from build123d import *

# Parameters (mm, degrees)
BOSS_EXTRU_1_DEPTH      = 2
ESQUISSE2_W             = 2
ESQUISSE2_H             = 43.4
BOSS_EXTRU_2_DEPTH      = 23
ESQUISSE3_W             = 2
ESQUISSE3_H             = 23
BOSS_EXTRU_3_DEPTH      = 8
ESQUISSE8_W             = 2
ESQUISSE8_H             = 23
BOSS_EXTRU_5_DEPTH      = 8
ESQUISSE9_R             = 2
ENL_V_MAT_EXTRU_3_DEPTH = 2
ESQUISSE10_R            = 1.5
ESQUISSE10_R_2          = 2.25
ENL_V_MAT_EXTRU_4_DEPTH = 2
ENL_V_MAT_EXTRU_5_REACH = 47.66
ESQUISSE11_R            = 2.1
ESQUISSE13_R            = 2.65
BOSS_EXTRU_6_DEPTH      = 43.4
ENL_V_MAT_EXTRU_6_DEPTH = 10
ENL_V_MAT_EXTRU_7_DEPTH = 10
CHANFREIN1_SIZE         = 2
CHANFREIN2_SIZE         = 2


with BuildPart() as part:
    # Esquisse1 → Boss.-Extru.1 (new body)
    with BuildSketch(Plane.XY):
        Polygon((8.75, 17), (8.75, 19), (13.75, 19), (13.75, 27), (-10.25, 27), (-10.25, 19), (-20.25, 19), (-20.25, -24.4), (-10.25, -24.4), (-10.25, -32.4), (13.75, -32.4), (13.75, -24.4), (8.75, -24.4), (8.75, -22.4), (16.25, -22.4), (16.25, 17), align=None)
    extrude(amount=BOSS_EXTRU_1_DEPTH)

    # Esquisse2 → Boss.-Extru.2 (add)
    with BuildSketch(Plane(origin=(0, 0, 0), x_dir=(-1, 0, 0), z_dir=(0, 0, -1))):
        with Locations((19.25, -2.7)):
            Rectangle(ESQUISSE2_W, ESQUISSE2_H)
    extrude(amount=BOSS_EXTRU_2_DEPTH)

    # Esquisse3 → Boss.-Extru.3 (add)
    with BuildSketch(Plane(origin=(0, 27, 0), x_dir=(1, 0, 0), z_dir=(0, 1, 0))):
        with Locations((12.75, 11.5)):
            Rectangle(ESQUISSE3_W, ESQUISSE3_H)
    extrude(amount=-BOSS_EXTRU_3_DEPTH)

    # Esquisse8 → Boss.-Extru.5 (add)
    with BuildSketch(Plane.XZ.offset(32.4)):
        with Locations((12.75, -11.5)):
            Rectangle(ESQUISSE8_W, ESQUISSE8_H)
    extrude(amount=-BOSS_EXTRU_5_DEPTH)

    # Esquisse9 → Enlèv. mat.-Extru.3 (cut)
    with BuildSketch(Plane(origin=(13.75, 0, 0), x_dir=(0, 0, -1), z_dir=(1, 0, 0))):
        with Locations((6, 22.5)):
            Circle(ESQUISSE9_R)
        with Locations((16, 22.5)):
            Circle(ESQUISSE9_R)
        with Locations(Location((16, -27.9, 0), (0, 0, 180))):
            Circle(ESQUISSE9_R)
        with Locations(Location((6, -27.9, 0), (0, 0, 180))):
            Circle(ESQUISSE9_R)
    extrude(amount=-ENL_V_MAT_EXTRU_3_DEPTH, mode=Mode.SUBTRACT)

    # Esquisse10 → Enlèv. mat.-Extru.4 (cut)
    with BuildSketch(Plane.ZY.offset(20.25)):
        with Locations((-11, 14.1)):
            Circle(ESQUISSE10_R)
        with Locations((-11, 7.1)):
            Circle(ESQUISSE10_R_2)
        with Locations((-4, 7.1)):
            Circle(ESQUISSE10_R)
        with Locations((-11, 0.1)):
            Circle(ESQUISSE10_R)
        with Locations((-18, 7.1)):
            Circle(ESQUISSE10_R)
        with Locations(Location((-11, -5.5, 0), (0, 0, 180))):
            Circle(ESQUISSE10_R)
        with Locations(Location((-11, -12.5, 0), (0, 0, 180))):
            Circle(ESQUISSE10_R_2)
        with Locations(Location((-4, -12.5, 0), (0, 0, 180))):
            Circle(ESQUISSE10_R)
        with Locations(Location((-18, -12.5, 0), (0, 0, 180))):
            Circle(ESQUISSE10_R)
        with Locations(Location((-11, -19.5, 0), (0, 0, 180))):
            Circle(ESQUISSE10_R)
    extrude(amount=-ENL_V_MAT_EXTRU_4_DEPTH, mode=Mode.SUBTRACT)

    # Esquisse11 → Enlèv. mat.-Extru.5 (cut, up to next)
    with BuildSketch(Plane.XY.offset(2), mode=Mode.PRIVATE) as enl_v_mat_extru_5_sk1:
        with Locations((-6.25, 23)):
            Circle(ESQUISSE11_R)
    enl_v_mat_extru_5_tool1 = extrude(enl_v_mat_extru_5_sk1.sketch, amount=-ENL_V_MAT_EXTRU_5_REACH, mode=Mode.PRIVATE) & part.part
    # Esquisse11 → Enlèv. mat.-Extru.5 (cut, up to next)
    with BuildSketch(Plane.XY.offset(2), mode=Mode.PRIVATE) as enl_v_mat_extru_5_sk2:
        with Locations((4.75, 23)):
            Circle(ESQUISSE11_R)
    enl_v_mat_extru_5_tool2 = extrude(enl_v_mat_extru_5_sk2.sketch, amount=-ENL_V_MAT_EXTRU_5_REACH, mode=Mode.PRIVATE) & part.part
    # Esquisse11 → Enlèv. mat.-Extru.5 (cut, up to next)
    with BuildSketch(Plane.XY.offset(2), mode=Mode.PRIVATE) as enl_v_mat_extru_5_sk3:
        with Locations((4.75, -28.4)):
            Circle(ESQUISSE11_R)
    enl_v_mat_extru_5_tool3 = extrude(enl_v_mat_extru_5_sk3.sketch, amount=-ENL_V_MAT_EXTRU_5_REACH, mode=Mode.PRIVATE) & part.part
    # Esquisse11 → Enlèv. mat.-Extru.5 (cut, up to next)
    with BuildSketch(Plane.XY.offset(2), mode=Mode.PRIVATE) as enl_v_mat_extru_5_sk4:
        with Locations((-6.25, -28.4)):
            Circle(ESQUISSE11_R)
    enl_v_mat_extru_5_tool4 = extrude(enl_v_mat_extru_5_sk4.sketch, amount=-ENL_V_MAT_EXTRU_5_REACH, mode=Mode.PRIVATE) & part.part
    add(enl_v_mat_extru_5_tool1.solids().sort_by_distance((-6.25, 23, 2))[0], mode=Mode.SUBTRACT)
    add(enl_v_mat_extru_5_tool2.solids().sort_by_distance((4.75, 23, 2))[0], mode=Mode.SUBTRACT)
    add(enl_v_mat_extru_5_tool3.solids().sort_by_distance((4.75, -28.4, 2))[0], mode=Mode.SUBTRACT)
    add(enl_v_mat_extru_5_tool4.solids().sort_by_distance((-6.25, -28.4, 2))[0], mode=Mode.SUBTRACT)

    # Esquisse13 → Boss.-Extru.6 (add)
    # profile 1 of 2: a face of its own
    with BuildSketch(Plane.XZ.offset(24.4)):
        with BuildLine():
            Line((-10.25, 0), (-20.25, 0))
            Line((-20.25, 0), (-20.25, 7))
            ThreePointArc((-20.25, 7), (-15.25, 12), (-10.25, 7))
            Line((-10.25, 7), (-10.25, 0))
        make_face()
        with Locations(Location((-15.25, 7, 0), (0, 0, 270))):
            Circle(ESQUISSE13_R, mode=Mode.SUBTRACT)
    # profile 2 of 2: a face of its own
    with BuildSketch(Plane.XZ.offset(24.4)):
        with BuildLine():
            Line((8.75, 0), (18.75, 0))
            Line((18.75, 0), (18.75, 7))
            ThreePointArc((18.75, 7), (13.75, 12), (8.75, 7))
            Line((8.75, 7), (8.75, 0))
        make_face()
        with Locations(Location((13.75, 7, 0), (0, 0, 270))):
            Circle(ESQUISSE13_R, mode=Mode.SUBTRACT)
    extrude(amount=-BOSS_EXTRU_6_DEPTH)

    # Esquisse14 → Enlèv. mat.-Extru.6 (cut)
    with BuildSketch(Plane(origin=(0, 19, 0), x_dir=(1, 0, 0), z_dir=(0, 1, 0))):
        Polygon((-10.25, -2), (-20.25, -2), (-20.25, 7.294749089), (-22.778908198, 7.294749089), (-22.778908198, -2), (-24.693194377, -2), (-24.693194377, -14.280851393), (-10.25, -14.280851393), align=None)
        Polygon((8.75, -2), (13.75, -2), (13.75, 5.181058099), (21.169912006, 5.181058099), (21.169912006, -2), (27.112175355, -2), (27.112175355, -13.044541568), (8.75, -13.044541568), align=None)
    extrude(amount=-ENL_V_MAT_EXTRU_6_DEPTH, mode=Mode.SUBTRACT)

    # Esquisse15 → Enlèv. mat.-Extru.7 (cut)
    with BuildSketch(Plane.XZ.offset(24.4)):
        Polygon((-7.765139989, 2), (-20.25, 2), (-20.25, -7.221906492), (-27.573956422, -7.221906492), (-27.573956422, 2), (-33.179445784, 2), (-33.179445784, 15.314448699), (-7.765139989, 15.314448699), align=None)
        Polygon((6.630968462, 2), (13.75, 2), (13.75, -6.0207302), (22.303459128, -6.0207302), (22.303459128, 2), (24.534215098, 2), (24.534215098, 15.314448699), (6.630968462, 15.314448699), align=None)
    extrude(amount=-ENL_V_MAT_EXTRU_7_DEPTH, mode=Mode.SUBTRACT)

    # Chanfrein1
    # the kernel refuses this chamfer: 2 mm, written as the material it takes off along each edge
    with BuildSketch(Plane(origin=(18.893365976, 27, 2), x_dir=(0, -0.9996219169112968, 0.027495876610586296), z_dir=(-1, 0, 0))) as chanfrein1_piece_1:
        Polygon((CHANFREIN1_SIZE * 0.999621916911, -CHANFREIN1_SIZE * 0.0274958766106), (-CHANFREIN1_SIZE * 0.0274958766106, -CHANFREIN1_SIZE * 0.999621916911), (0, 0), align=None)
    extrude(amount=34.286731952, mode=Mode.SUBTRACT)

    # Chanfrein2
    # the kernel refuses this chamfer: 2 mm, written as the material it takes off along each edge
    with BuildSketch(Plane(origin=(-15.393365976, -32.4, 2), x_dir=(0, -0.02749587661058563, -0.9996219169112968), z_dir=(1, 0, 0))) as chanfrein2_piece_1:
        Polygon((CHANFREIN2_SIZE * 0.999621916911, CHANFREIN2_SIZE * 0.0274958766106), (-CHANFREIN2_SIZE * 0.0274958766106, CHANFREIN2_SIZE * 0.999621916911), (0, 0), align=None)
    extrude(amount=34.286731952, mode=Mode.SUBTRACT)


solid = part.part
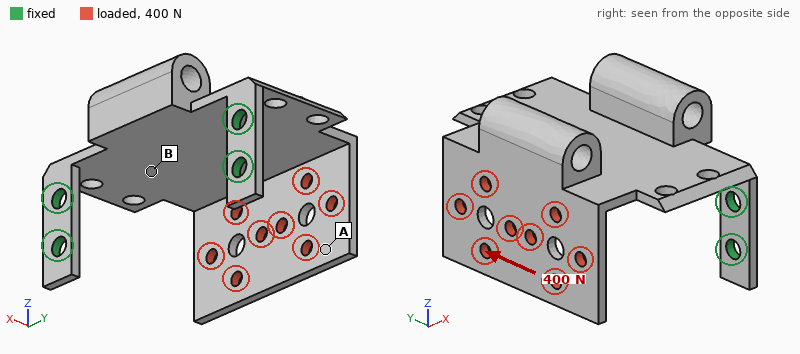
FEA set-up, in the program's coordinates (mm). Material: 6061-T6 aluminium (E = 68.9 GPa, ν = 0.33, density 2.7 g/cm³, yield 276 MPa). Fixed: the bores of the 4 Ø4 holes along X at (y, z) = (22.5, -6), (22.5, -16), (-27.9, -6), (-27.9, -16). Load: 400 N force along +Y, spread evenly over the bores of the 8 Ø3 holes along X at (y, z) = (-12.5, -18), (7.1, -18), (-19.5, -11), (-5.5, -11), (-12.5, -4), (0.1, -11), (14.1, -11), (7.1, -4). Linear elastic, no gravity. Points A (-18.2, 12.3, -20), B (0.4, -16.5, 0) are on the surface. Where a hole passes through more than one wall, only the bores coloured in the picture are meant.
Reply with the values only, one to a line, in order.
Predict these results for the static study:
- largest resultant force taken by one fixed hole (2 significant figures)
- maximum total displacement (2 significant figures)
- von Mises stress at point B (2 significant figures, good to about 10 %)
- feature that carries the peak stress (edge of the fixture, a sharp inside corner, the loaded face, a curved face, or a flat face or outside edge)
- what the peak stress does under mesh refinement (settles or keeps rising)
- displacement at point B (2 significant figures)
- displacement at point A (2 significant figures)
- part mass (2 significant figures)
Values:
360 N
0.65 mm
60 MPa
edge of the fixture
keeps rising
0.13 mm
0.54 mm
25 g
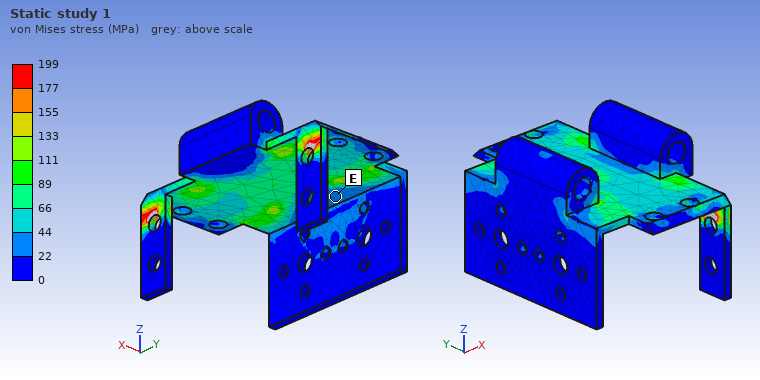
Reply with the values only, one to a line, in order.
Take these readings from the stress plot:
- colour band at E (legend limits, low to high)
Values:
22 to 44 MPa
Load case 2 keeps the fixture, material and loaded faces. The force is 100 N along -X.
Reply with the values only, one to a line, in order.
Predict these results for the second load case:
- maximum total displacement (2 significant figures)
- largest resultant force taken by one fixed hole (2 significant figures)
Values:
0.92 mm
51 N
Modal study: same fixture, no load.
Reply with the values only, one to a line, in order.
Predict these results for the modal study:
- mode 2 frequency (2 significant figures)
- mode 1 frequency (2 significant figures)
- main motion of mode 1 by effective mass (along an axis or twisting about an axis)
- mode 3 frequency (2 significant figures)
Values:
1600 Hz
360 Hz
along Z
1900 Hz
